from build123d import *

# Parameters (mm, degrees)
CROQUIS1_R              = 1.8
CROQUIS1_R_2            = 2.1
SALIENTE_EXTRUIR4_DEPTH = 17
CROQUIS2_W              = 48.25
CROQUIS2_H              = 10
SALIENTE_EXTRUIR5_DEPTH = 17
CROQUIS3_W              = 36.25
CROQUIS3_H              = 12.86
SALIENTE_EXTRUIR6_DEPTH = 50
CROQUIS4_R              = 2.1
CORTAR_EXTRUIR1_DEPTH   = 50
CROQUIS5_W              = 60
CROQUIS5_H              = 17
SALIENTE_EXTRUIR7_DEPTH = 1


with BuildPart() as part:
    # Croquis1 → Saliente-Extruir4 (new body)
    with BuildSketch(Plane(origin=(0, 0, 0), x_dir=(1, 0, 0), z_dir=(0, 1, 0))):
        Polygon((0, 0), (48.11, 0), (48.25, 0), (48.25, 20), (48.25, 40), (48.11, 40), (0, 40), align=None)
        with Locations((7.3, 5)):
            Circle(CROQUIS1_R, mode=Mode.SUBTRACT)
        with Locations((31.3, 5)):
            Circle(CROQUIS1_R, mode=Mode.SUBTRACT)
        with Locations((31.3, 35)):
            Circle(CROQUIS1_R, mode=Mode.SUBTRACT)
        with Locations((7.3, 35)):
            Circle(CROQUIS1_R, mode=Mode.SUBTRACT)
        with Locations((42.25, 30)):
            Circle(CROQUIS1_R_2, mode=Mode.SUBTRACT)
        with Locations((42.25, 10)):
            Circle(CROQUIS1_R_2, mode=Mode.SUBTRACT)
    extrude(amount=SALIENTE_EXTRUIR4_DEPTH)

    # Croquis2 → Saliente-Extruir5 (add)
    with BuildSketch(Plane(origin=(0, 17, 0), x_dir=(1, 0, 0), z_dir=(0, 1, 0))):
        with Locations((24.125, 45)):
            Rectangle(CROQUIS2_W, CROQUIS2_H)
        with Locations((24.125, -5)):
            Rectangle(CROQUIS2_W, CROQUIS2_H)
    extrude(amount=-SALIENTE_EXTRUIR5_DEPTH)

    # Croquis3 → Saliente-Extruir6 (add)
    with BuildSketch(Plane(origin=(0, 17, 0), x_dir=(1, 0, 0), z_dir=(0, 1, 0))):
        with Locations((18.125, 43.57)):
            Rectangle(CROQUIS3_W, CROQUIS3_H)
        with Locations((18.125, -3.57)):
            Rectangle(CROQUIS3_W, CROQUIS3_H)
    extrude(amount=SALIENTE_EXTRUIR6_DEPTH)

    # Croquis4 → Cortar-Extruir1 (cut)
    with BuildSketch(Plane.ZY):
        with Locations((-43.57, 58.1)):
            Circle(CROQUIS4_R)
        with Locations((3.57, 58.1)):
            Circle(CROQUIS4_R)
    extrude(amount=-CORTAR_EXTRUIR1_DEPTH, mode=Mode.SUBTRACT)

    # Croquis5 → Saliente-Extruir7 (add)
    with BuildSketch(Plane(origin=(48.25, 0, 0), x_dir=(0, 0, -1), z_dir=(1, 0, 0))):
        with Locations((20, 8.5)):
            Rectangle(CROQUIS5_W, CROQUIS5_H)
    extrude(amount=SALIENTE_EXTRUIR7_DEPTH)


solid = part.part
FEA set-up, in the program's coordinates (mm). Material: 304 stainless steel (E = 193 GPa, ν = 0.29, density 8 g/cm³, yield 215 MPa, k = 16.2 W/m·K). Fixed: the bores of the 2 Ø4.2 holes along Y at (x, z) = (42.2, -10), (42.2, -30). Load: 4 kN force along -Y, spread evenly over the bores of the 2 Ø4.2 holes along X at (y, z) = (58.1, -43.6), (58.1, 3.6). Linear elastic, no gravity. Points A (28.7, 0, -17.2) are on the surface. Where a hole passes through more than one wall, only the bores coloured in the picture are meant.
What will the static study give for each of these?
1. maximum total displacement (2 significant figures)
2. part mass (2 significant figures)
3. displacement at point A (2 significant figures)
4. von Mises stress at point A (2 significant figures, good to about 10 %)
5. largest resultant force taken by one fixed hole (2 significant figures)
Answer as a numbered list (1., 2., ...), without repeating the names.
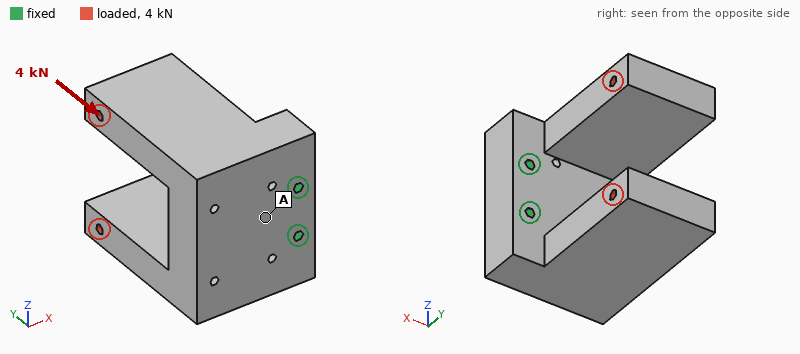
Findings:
1. 30 µm
2. 760 g
3. 4.8 µm
4. 17 MPa
5. 2.0 kN
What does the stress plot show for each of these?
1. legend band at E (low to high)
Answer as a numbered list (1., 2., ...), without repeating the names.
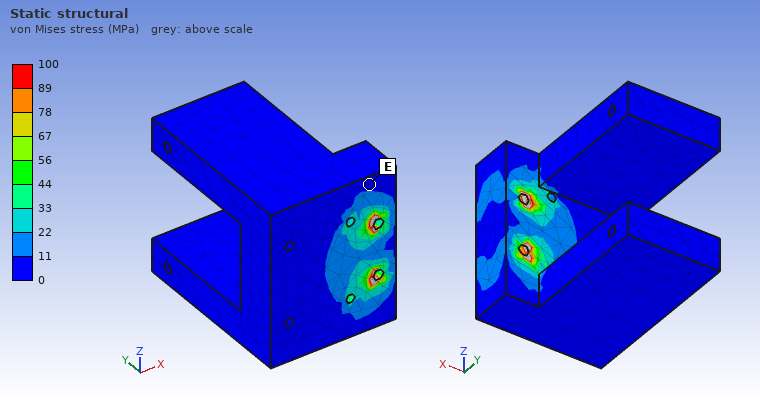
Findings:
1. 0 to 11 MPa
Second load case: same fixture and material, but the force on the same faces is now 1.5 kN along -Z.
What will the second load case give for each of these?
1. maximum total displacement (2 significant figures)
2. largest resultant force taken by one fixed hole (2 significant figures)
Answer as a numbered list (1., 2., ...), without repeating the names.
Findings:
1. 49 µm
2. 2.3 kN
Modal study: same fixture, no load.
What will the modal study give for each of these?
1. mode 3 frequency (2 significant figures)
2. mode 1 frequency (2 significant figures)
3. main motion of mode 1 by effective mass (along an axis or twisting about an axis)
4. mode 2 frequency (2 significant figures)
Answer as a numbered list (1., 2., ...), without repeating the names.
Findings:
1. 2700 Hz
2. 2300 Hz
3. along Z
4. 2400 Hz
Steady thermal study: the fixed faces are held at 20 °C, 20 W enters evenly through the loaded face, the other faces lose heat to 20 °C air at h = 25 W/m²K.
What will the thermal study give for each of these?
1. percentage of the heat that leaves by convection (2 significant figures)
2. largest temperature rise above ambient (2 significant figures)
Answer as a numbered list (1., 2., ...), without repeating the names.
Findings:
1. 59 %
2. 54 K
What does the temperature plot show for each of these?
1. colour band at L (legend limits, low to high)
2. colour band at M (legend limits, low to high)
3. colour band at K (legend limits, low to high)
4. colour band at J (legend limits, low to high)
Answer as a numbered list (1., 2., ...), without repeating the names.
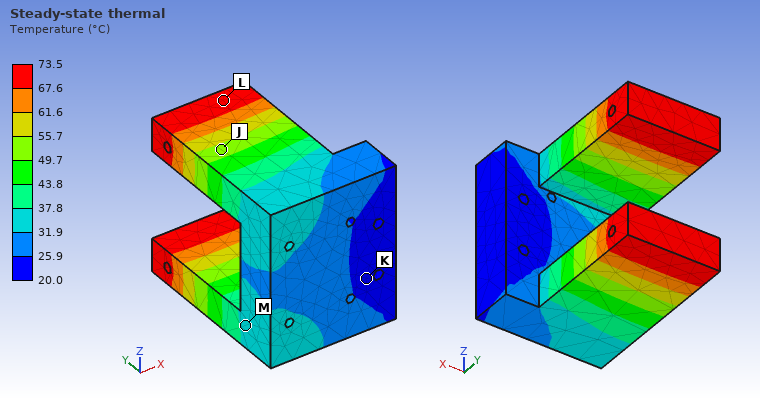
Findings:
1. 67.6 to 73.5 °C
2. 31.9 to 37.8 °C
3. 20.0 to 25.9 °C
4. 49.7 to 55.7 °C
